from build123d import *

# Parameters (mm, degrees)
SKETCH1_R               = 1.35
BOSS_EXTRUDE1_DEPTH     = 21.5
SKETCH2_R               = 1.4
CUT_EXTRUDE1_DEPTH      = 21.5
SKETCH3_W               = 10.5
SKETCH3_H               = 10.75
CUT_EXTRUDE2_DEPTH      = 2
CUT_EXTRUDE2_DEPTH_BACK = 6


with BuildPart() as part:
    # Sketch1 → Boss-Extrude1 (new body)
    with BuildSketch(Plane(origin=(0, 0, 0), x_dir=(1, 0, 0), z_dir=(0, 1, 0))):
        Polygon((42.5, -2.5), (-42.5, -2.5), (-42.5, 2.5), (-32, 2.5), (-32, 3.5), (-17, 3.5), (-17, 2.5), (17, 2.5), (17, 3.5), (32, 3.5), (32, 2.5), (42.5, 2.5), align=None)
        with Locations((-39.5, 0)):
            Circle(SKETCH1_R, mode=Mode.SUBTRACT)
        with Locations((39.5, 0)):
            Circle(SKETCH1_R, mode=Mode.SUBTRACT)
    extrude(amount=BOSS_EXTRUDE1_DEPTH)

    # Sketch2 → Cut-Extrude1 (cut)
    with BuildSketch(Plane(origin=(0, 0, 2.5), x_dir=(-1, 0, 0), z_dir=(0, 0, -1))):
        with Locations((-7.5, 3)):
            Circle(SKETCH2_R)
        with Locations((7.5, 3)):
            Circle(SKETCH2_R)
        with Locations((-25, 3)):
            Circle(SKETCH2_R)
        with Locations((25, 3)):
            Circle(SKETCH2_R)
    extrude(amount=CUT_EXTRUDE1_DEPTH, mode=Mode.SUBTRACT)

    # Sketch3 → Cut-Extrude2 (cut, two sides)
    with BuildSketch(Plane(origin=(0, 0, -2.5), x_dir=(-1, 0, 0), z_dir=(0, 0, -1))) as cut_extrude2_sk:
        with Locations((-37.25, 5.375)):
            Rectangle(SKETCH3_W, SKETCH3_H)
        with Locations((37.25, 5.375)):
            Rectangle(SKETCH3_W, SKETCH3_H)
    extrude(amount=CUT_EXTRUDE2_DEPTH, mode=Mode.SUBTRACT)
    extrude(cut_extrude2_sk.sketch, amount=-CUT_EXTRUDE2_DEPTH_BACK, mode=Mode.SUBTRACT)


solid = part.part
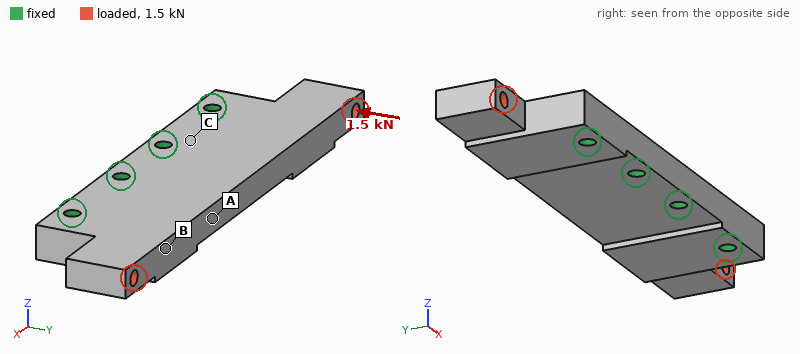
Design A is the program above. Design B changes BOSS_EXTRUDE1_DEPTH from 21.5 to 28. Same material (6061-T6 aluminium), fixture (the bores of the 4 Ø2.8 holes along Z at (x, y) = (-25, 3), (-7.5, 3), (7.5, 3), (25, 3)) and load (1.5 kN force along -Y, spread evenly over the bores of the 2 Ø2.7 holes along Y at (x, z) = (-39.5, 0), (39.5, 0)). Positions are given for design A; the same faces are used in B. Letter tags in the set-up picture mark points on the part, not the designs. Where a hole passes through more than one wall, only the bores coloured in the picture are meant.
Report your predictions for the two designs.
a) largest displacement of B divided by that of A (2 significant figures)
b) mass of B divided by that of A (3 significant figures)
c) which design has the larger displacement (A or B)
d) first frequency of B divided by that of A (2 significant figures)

0.54
1.34
A
0.61
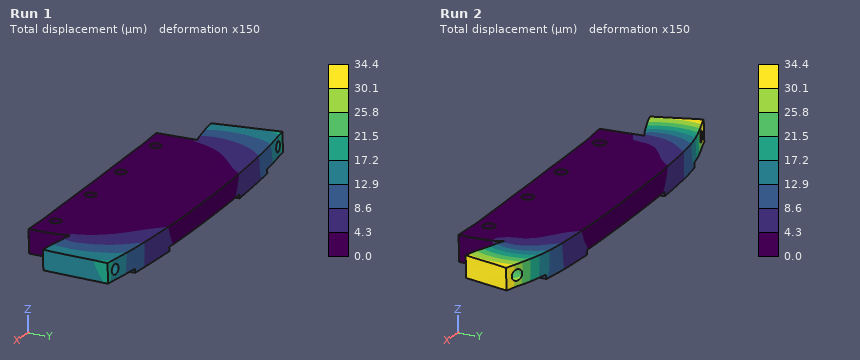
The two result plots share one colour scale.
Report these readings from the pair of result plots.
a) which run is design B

Run 1
